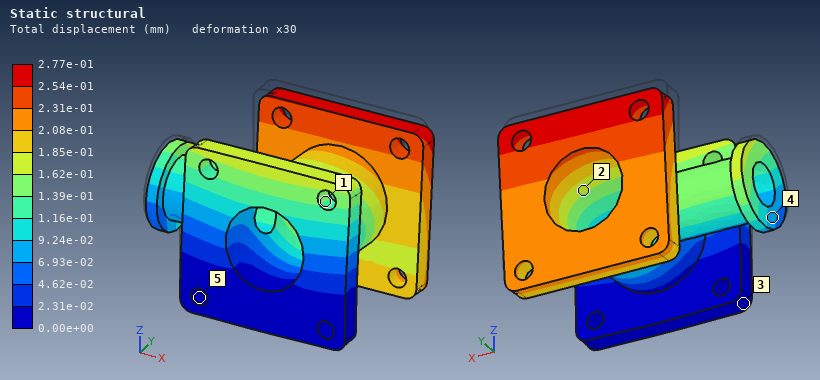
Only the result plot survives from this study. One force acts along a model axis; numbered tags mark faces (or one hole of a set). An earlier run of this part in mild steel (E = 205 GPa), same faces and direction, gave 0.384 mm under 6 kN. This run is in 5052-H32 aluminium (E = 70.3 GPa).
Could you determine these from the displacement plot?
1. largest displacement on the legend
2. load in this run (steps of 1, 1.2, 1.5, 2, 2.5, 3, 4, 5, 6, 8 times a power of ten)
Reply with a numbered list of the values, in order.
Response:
1. 2.77e-01 mm
2. 1.5 kN
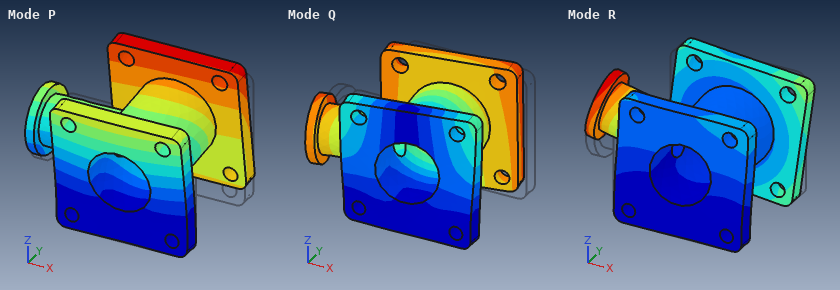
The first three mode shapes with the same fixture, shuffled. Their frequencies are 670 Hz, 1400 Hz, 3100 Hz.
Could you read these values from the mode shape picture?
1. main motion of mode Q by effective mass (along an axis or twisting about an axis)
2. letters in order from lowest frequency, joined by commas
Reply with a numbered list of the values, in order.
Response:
1. along X
2. P, Q, R
